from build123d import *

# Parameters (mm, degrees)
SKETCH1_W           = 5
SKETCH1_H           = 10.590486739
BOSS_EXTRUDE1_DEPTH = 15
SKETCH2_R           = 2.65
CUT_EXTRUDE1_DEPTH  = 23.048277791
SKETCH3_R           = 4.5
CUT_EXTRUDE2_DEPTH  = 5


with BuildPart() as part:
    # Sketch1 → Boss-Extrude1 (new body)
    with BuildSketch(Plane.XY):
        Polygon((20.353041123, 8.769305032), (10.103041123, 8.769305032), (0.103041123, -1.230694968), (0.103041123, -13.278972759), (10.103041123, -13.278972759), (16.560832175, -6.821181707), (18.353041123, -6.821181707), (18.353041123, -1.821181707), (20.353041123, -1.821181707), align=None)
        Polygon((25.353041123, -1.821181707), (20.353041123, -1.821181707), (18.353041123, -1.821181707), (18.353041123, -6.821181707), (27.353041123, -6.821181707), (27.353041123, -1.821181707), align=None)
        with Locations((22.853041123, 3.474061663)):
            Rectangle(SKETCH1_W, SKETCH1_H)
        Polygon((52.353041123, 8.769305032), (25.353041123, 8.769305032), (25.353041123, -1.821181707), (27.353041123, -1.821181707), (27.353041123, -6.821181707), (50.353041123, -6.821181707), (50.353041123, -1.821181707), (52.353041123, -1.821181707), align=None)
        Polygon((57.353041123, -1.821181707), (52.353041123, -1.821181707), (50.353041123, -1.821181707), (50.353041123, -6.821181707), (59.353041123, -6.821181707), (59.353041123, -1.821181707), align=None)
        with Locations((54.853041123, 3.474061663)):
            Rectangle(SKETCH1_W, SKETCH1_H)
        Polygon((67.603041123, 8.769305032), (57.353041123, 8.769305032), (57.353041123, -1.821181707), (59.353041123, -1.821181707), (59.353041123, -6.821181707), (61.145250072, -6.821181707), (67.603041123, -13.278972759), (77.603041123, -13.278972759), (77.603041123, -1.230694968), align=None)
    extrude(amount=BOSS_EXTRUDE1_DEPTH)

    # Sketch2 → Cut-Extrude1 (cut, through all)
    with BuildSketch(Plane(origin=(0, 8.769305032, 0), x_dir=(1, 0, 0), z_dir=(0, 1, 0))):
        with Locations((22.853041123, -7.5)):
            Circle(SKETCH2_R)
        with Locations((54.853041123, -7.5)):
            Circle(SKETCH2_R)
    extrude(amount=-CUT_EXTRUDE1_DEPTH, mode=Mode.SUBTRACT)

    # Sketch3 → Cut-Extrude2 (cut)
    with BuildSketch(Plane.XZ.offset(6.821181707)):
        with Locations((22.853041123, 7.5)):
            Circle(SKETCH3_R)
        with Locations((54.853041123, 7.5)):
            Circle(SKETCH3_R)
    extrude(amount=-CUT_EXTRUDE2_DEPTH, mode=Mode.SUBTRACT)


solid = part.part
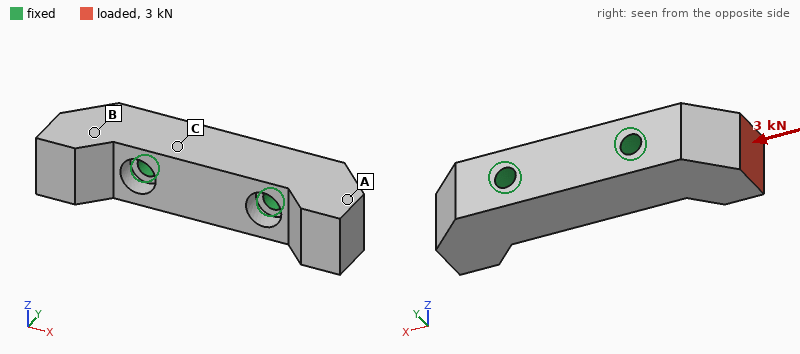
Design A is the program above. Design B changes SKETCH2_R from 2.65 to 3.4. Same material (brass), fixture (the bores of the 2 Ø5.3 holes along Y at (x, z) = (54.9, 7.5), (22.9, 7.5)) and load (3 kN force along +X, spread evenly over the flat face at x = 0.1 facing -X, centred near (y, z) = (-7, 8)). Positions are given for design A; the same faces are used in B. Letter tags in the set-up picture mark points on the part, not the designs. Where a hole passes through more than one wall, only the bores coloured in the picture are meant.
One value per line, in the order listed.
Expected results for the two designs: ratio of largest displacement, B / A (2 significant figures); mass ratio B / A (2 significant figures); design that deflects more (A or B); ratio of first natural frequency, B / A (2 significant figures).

0.89
0.98
A
1.1
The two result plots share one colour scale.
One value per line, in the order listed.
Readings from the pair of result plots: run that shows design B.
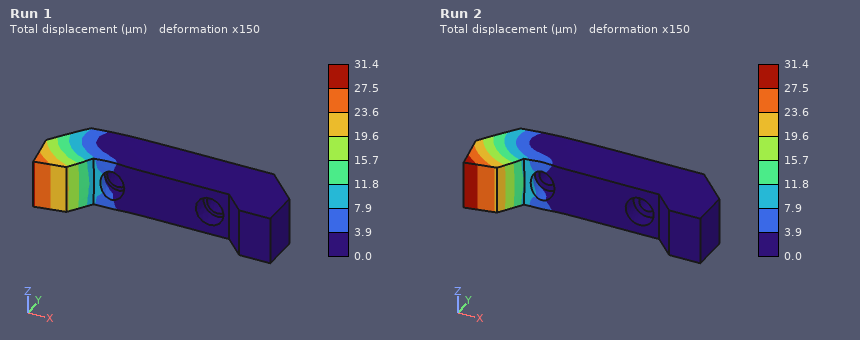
Run 1
